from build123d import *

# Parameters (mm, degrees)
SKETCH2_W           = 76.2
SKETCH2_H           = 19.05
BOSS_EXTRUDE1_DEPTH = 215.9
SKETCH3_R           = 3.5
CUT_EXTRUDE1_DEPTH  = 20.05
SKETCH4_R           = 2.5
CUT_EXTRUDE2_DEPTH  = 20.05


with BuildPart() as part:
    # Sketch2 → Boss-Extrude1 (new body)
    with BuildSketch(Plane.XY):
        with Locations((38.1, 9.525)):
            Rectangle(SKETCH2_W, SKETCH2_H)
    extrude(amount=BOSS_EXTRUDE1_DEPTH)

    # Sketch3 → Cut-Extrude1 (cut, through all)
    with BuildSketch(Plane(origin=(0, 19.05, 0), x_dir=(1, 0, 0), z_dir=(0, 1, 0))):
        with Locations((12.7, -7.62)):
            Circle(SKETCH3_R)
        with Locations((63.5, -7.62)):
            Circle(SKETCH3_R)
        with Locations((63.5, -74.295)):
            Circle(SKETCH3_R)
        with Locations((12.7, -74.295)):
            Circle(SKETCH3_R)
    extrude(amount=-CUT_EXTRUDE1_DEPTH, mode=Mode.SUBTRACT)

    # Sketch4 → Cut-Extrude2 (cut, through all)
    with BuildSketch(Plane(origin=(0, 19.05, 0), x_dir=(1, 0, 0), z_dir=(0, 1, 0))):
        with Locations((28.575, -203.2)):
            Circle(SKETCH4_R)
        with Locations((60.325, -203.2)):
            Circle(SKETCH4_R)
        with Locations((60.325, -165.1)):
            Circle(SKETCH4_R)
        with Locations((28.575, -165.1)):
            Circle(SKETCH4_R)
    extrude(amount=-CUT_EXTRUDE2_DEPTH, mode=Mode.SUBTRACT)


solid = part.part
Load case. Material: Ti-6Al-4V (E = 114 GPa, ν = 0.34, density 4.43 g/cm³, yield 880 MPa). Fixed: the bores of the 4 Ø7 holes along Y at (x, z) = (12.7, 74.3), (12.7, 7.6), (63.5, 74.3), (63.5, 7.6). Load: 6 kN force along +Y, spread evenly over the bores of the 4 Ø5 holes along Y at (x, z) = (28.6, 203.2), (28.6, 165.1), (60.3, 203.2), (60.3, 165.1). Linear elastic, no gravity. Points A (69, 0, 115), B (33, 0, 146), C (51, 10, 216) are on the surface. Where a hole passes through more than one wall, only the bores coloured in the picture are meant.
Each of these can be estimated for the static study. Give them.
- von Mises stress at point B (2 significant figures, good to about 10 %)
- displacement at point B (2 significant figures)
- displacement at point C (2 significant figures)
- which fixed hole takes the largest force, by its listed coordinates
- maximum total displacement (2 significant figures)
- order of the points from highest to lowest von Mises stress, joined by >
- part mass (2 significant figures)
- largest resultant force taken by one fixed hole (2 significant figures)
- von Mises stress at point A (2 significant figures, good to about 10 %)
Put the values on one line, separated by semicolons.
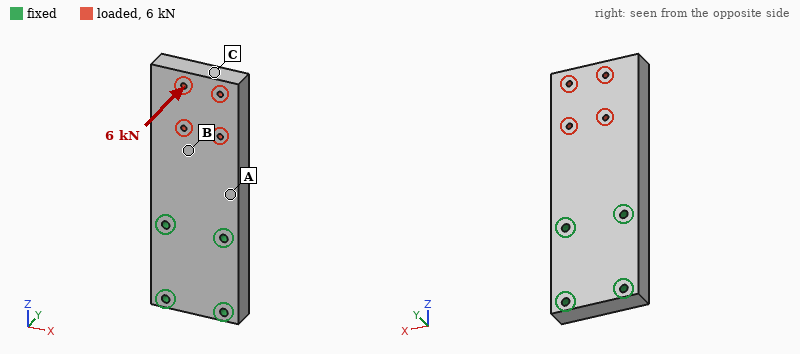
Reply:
51 MPa; 0.31 mm; 0.84 mm; (63.5, 74.3); 0.85 mm; A > B > C; 1.4 kg; 5.1 kN; 92 MPa
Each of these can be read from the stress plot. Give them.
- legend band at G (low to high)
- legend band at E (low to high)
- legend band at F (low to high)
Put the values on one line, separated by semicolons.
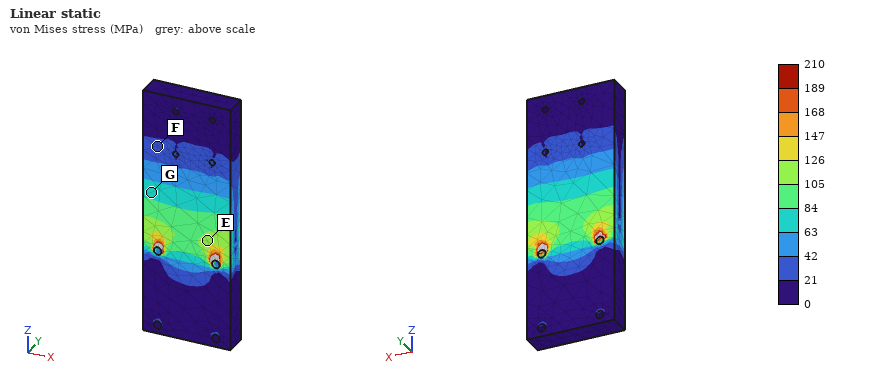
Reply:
63 to 84 MPa; 105 to 126 MPa; 21 to 42 MPa
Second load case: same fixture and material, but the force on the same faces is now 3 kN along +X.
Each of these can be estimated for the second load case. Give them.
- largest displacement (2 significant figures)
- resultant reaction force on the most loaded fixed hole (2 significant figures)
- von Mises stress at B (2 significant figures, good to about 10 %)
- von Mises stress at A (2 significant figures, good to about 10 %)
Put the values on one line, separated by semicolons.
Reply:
34 µm; 5.7 kN; 5.3 MPa; 9.3 MPa
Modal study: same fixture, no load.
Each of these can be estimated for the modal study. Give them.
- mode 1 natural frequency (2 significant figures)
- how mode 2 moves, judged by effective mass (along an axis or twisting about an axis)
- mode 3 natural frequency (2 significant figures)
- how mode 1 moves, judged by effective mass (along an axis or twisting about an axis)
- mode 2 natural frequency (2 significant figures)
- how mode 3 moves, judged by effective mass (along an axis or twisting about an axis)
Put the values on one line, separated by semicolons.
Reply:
750 Hz; along X; 2700 Hz; along Y; 2500 Hz; twisting about Z
